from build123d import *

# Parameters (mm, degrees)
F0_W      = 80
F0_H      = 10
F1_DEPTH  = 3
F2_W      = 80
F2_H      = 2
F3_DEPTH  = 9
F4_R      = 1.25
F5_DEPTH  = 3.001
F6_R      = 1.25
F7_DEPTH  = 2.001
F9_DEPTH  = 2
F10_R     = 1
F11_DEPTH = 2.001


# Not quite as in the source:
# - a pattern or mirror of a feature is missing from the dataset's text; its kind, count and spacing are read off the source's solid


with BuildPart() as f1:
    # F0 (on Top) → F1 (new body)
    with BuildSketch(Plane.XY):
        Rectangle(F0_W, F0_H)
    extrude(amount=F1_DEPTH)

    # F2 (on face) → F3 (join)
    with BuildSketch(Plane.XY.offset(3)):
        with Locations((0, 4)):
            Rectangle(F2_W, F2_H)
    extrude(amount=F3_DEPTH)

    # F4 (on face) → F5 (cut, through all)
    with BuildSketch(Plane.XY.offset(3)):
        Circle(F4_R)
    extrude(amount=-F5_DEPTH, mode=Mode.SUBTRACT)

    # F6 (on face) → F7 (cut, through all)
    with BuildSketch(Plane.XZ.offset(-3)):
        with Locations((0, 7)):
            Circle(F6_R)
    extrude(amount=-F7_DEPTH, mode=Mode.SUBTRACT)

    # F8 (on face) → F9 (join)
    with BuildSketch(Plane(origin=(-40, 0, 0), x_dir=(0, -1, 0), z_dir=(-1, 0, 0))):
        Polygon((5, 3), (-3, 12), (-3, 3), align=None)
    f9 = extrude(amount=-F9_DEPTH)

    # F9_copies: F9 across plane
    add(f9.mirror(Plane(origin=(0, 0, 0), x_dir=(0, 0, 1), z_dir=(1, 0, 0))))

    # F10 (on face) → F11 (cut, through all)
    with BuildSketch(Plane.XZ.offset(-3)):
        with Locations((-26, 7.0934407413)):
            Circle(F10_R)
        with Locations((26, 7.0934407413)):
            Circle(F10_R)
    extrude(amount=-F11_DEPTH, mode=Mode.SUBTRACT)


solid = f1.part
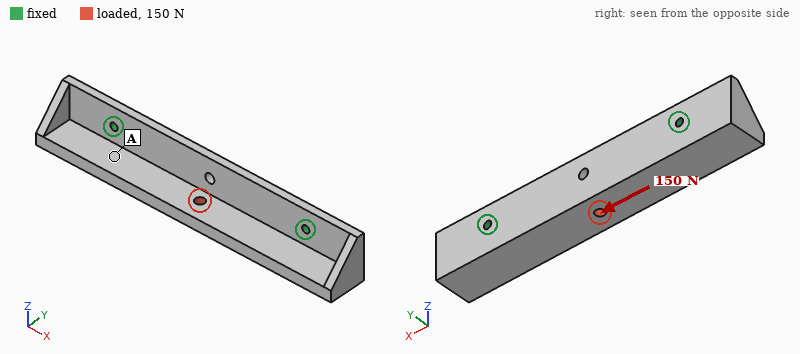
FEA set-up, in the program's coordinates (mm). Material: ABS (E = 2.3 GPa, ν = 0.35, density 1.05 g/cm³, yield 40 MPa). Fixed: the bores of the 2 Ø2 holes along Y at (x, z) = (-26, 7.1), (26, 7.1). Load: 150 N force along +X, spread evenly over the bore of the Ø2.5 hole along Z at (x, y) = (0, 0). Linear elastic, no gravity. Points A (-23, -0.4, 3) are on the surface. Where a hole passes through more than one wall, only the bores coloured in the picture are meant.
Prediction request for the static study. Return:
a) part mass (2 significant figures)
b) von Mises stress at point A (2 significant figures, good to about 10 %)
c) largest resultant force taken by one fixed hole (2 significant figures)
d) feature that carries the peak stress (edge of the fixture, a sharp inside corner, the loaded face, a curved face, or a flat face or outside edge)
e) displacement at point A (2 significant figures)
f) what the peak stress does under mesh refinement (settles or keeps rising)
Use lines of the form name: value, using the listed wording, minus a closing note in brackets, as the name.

part mass: 4.1 g
von Mises stress at point A: 1.7 MPa
largest resultant force taken by one fixed hole: 77 N
feature that carries the peak stress: edge of the fixture
displacement at point A: 34 µm
what the peak stress does under mesh refinement: keeps rising
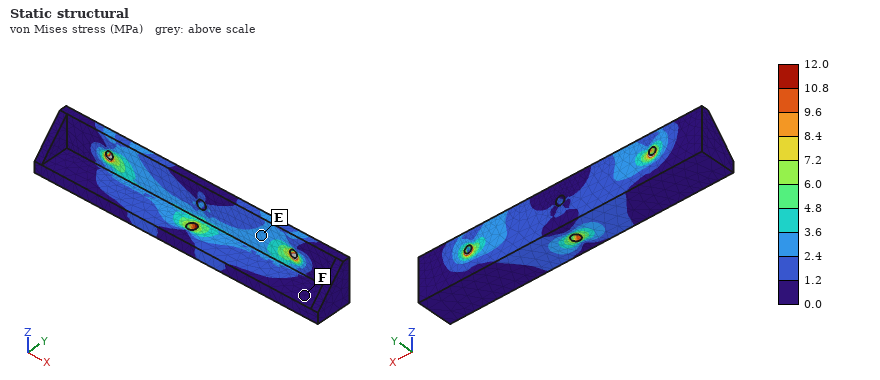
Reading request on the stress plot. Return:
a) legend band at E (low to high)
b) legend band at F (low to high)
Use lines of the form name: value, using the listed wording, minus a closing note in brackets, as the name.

legend band at E: 2.4 to 3.6 MPa
legend band at F: 0.0 to 1.2 MPa
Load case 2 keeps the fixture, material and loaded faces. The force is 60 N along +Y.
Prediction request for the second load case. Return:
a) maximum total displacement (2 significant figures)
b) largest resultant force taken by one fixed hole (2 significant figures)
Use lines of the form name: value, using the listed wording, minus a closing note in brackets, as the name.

maximum total displacement: 0.45 mm
largest resultant force taken by one fixed hole: 40 N
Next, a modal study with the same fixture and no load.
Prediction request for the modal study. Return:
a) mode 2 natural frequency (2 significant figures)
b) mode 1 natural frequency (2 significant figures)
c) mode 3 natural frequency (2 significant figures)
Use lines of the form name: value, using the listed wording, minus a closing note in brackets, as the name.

mode 2 natural frequency: 2000 Hz
mode 1 natural frequency: 1500 Hz
mode 3 natural frequency: 2200 Hz
